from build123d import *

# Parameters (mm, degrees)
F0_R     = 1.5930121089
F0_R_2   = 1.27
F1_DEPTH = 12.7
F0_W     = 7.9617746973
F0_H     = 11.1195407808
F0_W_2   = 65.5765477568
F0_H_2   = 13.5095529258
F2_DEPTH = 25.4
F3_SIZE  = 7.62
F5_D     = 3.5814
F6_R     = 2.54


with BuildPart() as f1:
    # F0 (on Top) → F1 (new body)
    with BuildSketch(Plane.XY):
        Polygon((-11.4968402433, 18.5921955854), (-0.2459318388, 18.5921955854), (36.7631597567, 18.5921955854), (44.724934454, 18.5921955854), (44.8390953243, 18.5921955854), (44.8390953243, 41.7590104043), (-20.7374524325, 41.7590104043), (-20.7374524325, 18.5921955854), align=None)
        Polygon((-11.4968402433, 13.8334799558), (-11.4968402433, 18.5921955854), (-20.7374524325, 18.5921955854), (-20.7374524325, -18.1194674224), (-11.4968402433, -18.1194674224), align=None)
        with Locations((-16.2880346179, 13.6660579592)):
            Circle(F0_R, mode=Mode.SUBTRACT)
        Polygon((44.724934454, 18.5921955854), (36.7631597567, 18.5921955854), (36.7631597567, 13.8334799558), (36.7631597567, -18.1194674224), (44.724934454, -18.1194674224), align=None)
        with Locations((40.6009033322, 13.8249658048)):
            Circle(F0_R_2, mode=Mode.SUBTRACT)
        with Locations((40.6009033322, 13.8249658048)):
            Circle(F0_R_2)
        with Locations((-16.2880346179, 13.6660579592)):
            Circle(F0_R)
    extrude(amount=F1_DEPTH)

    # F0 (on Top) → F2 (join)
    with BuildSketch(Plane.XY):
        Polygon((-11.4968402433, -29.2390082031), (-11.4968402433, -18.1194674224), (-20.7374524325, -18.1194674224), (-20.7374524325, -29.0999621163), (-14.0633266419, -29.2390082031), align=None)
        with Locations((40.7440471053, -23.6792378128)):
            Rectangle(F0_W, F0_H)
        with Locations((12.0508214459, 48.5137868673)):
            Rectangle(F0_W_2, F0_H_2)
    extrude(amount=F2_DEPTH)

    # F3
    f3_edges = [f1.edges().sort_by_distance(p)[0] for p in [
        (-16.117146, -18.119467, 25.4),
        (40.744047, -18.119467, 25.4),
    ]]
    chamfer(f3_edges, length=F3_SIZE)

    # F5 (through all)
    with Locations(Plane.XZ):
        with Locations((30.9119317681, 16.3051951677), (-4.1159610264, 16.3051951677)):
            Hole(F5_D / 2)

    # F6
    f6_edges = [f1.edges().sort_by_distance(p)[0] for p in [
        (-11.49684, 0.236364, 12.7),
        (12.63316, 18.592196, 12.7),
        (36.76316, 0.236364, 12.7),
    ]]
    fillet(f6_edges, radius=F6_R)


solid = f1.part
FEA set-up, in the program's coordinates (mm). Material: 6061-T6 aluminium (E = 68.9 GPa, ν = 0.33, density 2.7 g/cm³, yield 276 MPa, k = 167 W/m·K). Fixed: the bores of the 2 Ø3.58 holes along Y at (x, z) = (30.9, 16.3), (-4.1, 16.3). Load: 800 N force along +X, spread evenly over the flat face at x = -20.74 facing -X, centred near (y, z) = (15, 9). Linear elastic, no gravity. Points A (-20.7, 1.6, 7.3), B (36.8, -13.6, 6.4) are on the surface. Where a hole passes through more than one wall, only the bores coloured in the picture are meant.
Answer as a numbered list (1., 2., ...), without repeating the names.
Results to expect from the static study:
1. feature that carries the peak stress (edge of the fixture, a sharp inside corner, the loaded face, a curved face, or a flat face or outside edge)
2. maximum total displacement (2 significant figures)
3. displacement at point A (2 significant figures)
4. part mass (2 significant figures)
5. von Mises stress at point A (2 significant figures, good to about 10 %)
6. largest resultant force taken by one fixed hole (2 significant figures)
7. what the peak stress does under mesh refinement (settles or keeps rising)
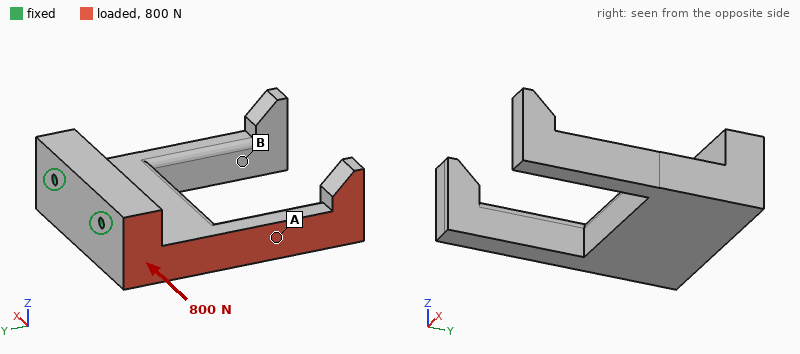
1. a sharp inside corner
2. 0.22 mm
3. 0.063 mm
4. 150 g
5. 30 MPa
6. 760 N
7. keeps rising
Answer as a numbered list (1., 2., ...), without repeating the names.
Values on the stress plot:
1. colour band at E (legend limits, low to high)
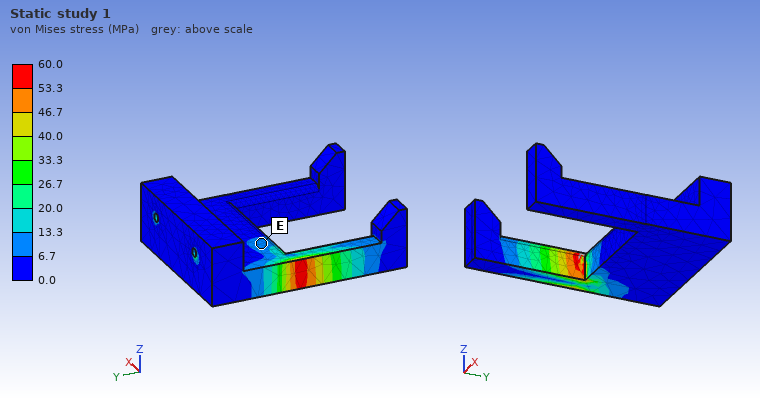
1. 6.7 to 13.3 MPa
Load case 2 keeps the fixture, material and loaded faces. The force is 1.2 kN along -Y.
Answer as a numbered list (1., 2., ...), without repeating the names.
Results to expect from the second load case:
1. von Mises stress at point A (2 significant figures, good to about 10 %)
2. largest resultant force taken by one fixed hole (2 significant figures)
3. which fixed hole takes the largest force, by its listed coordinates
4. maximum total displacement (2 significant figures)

1. 16 MPa
2. 1.5 kN
3. (-4.1, 16.3)
4. 83 µm
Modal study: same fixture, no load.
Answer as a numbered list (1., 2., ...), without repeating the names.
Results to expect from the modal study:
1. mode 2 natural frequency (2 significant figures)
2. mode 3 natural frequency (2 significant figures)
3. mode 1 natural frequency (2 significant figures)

1. 1800 Hz
2. 2000 Hz
3. 1800 Hz
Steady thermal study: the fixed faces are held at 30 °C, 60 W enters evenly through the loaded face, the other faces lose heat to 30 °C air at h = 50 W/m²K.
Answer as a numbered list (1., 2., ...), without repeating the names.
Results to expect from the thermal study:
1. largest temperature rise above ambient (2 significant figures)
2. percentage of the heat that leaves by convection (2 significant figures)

1. 64 K
2. 13 %
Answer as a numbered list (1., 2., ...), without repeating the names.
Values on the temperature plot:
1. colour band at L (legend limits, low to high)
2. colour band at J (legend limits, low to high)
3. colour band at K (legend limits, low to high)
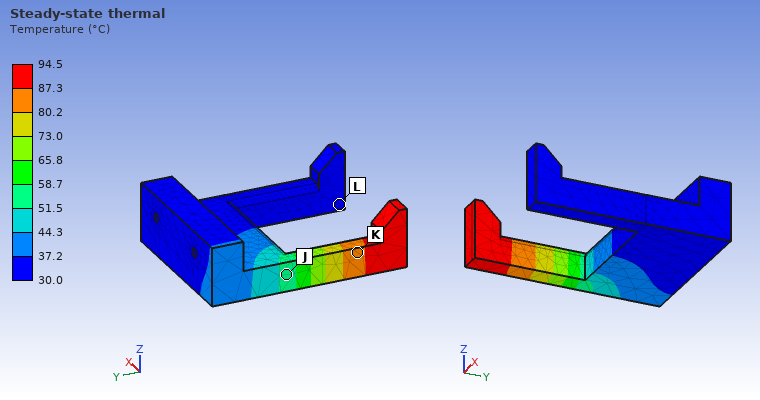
1. 30.0 to 37.2 °C
2. 51.5 to 58.7 °C
3. 80.2 to 87.3 °C
